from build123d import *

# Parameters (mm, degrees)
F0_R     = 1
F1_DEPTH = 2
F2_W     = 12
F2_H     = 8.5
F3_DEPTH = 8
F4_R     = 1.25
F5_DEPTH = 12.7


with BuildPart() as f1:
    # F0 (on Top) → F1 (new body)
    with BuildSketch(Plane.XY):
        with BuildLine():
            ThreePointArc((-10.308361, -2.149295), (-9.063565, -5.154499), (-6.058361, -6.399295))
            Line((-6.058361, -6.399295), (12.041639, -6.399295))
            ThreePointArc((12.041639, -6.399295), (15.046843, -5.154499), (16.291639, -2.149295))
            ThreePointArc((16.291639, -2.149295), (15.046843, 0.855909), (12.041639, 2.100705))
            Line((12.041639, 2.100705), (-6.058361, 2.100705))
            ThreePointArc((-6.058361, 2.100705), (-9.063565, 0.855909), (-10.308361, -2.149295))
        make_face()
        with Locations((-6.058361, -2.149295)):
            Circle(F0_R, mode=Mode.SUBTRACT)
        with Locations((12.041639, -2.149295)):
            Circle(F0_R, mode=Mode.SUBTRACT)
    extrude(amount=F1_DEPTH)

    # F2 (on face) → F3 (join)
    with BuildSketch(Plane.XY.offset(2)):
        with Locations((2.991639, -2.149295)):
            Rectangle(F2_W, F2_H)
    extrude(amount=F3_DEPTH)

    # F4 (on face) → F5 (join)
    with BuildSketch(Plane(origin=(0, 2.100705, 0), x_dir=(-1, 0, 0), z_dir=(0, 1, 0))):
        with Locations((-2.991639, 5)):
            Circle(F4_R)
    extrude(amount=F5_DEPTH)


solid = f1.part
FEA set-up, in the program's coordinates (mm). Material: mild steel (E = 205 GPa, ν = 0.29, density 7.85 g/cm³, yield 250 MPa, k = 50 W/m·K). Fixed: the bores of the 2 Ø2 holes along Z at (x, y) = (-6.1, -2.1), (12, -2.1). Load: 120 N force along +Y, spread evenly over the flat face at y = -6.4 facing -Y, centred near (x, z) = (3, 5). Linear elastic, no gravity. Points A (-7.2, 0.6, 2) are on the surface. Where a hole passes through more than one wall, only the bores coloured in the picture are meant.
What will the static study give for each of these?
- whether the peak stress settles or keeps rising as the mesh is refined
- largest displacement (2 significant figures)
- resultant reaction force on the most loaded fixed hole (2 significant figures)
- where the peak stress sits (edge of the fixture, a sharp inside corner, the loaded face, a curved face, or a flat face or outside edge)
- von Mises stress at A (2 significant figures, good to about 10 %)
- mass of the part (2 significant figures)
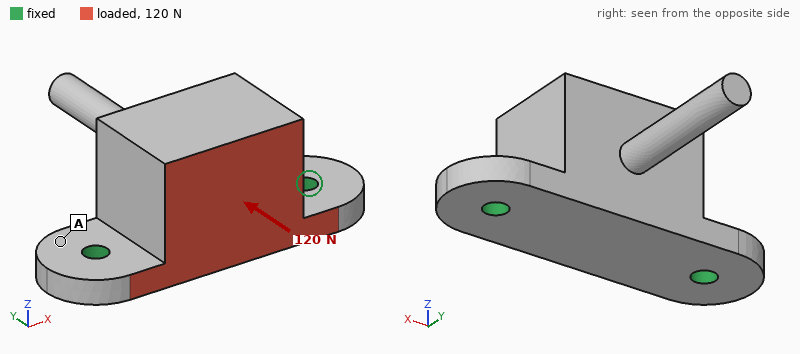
keeps rising
6.9 µm
60 N
edge of the fixture
11 MPa
10 g
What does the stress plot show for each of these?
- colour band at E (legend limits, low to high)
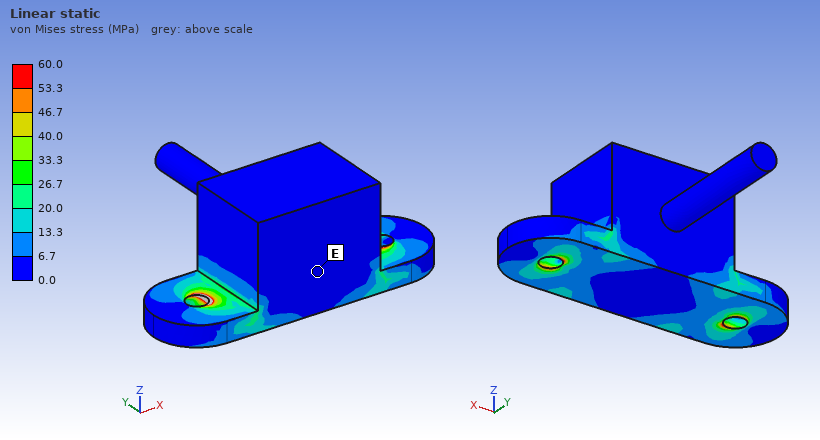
0.0 to 6.7 MPa
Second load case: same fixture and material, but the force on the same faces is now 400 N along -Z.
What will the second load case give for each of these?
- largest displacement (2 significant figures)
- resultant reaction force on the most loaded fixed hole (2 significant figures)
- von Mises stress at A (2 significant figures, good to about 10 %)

23 µm
220 N
33 MPa
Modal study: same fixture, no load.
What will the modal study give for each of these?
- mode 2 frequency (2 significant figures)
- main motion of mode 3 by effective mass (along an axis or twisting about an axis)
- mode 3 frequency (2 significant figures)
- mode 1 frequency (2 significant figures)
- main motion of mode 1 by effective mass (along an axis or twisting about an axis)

9900 Hz
along Y
12 kHz
8100 Hz
along Y
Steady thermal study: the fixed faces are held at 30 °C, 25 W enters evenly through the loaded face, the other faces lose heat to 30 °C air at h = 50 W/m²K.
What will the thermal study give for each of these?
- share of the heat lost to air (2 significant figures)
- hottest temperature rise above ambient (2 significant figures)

8.1 %
85 K
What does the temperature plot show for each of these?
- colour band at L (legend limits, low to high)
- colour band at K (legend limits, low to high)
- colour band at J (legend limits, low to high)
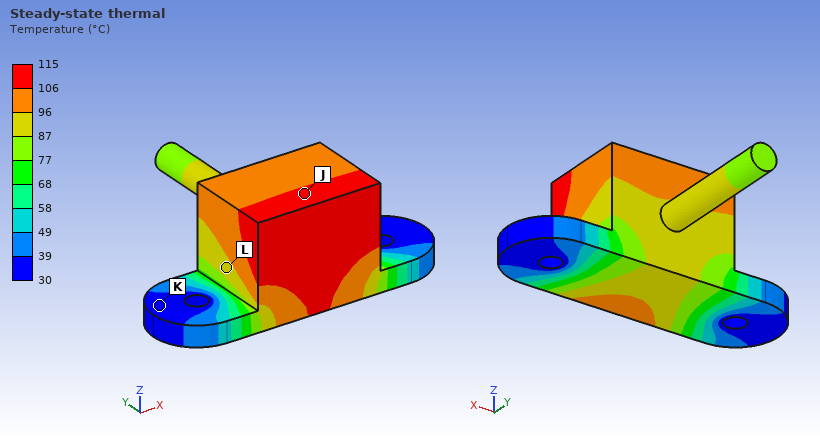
87 to 96 °C
30 to 39 °C
106 to 115 °C
